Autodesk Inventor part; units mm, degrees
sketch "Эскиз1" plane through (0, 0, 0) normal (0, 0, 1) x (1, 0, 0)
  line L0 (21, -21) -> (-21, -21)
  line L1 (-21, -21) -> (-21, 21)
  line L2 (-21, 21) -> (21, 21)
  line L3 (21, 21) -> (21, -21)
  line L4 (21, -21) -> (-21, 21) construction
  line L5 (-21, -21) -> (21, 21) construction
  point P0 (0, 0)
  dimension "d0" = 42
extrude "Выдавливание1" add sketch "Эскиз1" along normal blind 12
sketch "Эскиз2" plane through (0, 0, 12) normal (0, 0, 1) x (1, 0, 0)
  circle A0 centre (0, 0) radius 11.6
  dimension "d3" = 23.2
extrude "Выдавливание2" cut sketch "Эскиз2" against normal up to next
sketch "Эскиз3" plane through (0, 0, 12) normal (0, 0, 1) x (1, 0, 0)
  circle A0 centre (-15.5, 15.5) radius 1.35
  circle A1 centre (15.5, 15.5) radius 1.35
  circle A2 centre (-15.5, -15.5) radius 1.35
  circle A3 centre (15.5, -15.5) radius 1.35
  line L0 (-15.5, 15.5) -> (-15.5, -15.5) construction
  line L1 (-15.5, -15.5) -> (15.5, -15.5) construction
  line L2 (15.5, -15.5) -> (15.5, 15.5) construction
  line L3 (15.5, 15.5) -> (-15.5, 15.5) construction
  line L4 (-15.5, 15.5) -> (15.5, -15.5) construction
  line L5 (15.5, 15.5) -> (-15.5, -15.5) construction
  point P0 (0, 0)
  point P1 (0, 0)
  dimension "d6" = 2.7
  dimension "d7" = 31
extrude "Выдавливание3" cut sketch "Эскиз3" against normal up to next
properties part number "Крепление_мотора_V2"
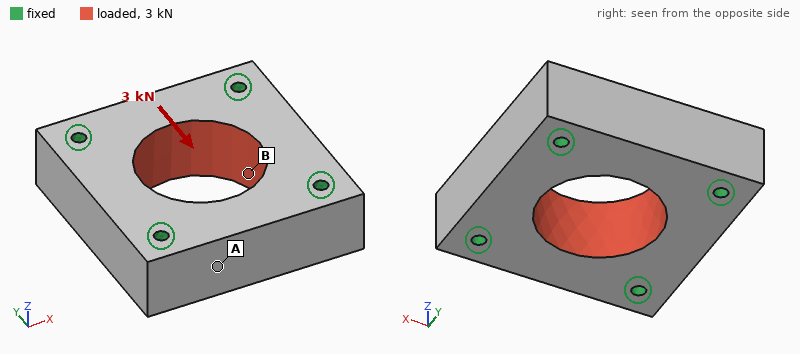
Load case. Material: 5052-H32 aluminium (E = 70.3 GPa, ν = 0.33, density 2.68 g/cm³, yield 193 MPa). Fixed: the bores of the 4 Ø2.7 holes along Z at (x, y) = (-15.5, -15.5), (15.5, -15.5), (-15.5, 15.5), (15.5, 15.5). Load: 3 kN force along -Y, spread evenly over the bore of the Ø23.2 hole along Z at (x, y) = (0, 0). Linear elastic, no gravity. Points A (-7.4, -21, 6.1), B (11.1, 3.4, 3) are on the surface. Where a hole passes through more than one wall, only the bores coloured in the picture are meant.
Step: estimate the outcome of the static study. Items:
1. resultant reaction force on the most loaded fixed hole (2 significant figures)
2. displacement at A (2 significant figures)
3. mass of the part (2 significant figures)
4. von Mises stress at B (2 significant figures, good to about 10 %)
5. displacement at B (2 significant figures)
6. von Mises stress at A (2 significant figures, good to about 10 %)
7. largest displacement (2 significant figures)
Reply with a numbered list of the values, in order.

1. 770 N
2. 1.6 µm
3. 42 g
4. 7.2 MPa
5. 1.0 µm
6. 3.2 MPa
7. 2.5 µm
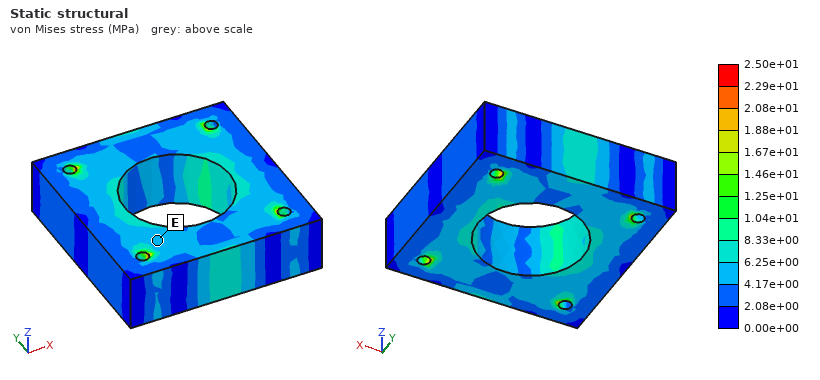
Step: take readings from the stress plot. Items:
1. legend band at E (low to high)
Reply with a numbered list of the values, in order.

1. 4.17e+00 to 6.25e+00 MPa
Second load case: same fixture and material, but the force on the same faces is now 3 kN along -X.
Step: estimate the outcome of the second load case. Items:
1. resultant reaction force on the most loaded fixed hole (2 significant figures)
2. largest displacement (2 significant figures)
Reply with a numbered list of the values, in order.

1. 770 N
2. 2.6 µm
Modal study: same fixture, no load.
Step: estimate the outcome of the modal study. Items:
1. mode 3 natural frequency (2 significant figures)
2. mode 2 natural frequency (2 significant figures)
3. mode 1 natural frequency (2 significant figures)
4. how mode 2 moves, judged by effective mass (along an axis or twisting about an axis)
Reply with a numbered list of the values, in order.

1. 38 kHz
2. 35 kHz
3. 26 kHz
4. along Z
